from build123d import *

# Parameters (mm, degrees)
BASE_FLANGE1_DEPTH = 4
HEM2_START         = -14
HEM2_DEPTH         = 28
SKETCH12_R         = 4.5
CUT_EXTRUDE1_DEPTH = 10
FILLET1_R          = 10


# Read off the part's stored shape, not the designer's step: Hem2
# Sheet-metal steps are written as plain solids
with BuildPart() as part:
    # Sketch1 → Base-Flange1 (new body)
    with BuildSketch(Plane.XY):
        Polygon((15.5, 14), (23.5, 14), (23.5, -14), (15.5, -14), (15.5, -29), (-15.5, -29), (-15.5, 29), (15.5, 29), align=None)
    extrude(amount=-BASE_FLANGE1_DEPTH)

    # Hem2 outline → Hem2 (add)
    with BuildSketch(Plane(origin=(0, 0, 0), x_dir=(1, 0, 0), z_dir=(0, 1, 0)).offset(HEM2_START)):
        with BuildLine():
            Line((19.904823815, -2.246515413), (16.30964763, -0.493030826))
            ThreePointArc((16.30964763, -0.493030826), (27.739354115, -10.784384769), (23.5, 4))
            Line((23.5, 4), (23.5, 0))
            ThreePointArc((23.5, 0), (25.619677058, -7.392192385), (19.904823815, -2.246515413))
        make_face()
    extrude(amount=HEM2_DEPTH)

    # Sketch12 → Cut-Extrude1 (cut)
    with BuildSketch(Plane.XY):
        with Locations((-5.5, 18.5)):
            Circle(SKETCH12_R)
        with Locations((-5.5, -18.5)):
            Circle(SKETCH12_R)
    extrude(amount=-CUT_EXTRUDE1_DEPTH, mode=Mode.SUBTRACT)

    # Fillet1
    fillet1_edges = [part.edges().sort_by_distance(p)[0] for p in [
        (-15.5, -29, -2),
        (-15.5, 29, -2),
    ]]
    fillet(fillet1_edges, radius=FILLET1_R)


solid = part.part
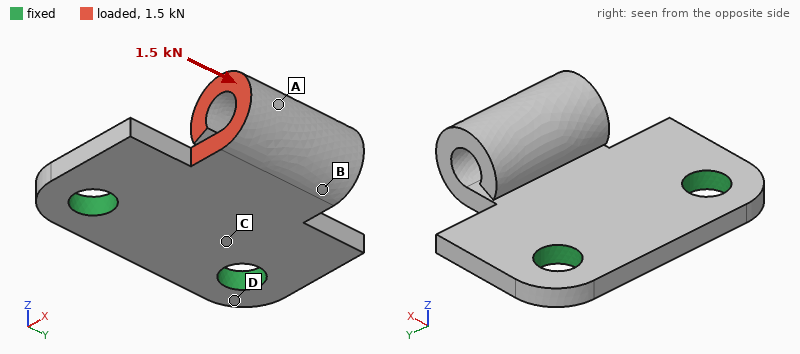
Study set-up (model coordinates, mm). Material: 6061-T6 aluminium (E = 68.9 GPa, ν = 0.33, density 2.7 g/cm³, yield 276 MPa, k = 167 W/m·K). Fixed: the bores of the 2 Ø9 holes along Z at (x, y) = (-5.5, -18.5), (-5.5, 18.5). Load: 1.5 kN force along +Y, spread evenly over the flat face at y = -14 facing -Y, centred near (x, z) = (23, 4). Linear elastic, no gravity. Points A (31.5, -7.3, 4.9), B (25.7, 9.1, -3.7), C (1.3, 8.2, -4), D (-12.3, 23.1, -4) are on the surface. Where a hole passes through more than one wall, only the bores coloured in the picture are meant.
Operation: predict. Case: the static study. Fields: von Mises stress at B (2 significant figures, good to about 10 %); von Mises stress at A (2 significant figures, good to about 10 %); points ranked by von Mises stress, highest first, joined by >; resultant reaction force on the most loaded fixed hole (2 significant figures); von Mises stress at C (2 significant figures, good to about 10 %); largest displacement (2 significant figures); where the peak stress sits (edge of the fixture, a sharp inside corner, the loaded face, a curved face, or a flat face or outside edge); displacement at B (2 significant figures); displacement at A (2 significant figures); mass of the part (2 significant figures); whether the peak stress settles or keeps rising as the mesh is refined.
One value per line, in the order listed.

64 MPa
47 MPa
B > A > C > D
1.3 kN
25 MPa
0.22 mm
a sharp inside corner
0.078 mm
0.11 mm
29 g
keeps rising
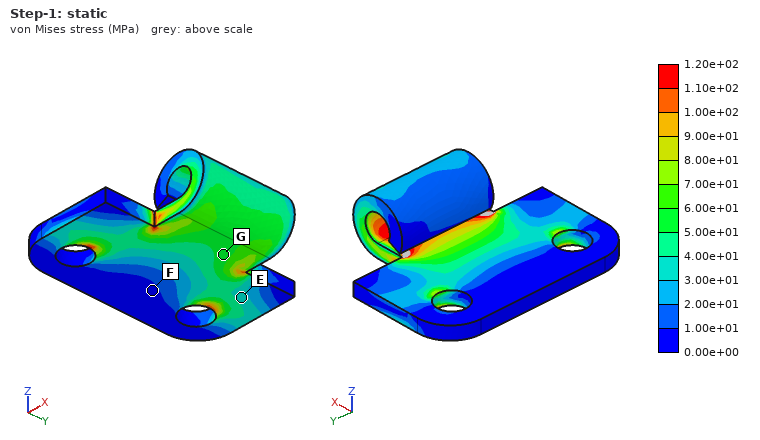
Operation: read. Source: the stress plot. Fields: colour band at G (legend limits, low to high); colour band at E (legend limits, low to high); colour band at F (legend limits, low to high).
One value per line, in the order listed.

5.00e+01 to 6.00e+01 MPa
3.00e+01 to 4.00e+01 MPa
0.00e+00 to 1.00e+01 MPa
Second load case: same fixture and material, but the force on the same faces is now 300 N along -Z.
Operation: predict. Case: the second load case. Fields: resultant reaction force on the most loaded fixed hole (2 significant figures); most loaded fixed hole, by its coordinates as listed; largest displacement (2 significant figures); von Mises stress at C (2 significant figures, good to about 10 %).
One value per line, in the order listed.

280 N
(-5.5, -18.5)
0.23 mm
30 MPa
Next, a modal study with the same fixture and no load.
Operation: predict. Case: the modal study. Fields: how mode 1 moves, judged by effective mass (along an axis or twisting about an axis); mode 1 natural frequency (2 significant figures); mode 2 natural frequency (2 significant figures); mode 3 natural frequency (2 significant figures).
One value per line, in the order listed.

along Z
2000 Hz
3900 Hz
4700 Hz
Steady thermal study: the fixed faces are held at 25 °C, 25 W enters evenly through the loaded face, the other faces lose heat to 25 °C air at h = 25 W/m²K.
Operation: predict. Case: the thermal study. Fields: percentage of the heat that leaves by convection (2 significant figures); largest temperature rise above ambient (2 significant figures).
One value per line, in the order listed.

9.9 %
49 K
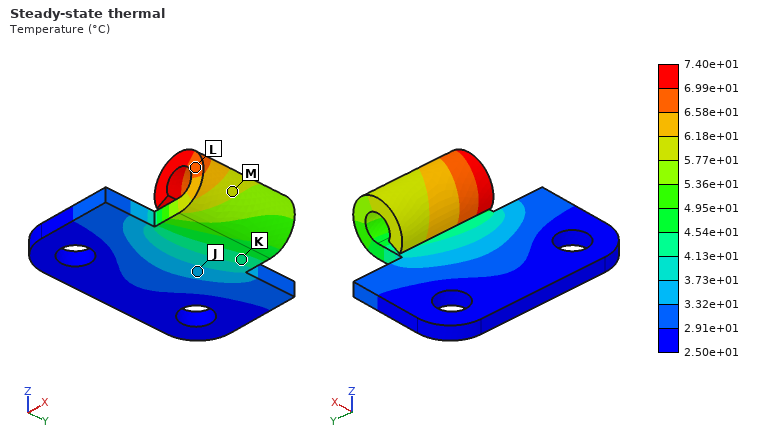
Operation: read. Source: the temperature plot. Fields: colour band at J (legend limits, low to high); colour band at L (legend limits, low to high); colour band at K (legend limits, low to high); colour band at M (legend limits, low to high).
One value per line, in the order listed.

3.32e+01 to 3.73e+01 °C
6.58e+01 to 6.99e+01 °C
4.13e+01 to 4.54e+01 °C
5.77e+01 to 6.18e+01 °C
